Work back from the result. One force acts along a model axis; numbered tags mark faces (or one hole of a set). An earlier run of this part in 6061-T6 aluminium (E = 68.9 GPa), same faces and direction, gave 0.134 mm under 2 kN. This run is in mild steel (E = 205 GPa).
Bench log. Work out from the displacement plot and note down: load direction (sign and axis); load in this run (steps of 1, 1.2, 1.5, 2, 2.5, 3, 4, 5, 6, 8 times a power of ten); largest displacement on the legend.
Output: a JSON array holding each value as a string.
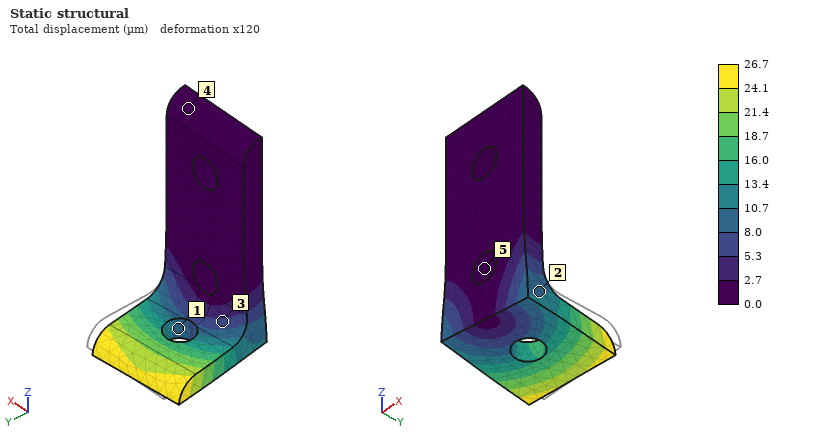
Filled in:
["-X", "1.2 kN", "26.7 µm"]
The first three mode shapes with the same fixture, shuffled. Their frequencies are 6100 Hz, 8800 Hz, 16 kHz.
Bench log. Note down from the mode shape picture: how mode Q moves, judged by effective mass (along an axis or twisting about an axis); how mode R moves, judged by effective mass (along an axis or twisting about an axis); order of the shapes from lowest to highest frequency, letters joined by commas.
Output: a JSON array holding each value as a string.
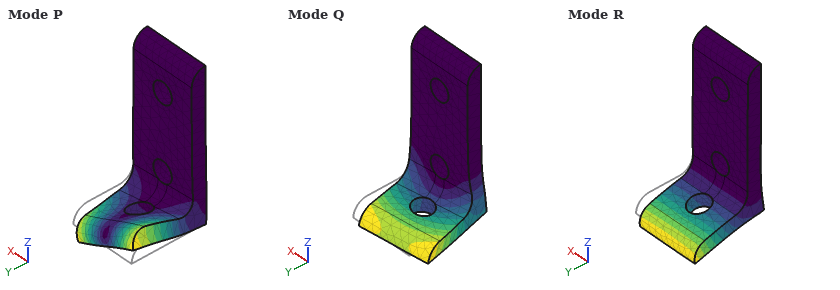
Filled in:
["along X", "along Z", "R, Q, P"]
